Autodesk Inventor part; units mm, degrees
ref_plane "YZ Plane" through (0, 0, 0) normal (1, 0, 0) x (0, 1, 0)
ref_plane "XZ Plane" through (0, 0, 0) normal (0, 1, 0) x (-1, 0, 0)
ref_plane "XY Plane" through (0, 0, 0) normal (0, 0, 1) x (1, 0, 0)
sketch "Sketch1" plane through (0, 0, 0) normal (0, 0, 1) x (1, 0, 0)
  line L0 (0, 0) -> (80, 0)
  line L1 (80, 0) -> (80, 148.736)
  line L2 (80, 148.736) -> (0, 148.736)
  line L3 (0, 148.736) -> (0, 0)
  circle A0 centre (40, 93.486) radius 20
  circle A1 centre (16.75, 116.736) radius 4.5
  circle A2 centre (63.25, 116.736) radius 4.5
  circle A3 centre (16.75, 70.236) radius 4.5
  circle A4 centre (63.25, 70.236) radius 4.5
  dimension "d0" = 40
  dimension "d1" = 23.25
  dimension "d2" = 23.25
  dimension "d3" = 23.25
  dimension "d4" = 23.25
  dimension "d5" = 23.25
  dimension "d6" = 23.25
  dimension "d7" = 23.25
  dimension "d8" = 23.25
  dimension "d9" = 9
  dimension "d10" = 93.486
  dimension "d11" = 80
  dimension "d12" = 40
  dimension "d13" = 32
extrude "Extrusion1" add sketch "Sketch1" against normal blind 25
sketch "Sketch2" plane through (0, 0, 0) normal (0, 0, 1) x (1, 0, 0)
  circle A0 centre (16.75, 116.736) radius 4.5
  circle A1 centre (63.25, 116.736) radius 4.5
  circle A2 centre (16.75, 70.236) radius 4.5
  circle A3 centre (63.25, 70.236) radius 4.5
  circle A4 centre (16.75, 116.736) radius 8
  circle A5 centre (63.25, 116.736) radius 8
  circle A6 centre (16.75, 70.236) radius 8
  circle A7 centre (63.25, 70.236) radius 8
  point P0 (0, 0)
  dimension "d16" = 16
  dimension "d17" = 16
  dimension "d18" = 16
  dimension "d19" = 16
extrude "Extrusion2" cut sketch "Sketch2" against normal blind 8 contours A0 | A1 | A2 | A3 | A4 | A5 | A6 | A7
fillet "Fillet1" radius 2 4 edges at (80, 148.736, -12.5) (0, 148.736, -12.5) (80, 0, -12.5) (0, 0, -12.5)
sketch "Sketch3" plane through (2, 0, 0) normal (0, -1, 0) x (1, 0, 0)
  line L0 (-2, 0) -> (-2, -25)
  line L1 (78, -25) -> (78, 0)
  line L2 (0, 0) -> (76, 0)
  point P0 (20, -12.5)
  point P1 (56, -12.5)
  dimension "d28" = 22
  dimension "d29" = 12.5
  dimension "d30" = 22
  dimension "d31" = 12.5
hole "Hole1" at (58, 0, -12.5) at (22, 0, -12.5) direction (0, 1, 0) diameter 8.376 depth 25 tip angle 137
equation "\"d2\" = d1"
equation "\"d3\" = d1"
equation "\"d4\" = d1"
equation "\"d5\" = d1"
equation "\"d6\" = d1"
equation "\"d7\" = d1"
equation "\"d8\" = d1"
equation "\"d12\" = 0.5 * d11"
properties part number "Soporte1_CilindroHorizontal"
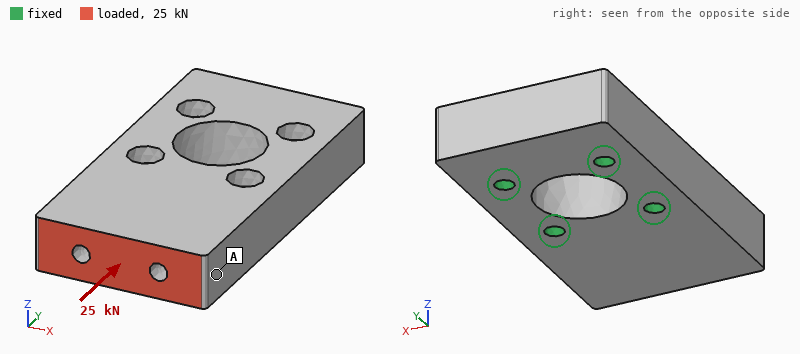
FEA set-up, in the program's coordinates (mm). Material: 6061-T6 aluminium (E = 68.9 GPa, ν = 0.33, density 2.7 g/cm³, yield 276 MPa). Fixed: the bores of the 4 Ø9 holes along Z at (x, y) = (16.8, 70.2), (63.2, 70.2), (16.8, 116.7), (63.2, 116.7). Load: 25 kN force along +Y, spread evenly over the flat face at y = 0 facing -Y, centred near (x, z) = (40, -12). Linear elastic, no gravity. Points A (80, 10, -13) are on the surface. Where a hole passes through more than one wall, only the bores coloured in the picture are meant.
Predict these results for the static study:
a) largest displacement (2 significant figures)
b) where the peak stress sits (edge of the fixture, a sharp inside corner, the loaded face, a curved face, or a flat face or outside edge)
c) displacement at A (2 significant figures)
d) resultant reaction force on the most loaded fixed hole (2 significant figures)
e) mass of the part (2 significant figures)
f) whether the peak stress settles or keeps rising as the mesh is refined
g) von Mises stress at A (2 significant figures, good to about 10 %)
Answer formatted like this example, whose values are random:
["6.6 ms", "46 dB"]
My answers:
["29 µm", "edge of the fixture", "21 µm", "11 kN", "680 g", "keeps rising", "8.2 MPa"]
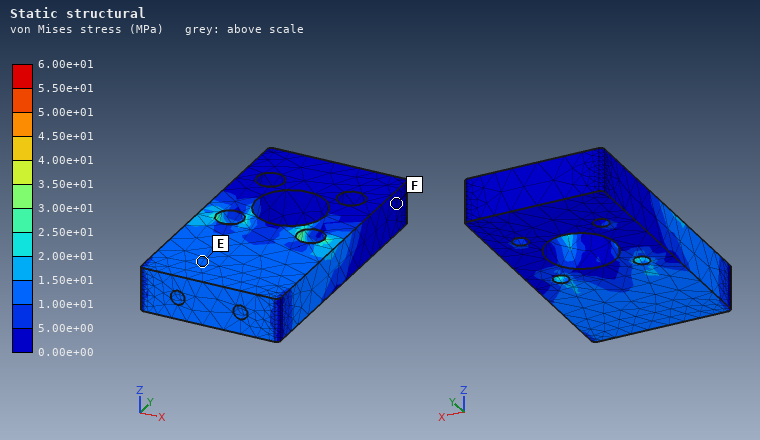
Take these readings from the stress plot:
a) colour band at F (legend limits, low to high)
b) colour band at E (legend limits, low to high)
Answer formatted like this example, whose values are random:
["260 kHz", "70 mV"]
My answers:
["0.00e+00 to 5.00e+00 MPa", "1.00e+01 to 1.50e+01 MPa"]
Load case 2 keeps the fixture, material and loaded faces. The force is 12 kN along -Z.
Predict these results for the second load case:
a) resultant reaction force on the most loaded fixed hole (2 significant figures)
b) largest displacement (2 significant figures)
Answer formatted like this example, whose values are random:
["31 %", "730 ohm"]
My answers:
["9.5 kN", "0.35 mm"]
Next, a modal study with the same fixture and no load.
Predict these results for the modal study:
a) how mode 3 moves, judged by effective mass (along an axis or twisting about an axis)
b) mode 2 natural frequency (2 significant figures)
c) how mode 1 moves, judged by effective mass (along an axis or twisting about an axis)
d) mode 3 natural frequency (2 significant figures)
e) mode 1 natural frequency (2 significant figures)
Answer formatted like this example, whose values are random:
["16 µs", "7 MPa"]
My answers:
["along X", "6400 Hz", "along Z", "7000 Hz", "2900 Hz"]
